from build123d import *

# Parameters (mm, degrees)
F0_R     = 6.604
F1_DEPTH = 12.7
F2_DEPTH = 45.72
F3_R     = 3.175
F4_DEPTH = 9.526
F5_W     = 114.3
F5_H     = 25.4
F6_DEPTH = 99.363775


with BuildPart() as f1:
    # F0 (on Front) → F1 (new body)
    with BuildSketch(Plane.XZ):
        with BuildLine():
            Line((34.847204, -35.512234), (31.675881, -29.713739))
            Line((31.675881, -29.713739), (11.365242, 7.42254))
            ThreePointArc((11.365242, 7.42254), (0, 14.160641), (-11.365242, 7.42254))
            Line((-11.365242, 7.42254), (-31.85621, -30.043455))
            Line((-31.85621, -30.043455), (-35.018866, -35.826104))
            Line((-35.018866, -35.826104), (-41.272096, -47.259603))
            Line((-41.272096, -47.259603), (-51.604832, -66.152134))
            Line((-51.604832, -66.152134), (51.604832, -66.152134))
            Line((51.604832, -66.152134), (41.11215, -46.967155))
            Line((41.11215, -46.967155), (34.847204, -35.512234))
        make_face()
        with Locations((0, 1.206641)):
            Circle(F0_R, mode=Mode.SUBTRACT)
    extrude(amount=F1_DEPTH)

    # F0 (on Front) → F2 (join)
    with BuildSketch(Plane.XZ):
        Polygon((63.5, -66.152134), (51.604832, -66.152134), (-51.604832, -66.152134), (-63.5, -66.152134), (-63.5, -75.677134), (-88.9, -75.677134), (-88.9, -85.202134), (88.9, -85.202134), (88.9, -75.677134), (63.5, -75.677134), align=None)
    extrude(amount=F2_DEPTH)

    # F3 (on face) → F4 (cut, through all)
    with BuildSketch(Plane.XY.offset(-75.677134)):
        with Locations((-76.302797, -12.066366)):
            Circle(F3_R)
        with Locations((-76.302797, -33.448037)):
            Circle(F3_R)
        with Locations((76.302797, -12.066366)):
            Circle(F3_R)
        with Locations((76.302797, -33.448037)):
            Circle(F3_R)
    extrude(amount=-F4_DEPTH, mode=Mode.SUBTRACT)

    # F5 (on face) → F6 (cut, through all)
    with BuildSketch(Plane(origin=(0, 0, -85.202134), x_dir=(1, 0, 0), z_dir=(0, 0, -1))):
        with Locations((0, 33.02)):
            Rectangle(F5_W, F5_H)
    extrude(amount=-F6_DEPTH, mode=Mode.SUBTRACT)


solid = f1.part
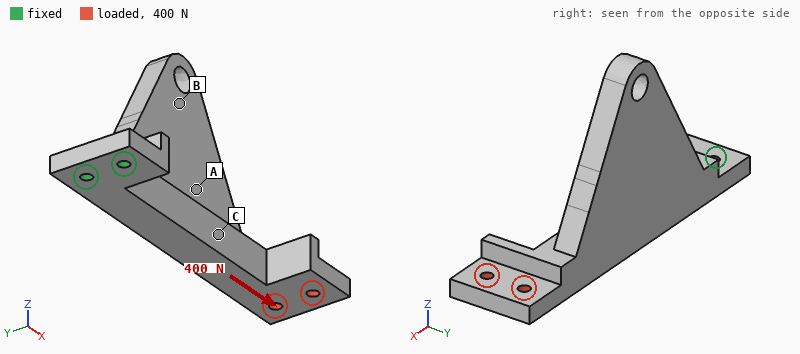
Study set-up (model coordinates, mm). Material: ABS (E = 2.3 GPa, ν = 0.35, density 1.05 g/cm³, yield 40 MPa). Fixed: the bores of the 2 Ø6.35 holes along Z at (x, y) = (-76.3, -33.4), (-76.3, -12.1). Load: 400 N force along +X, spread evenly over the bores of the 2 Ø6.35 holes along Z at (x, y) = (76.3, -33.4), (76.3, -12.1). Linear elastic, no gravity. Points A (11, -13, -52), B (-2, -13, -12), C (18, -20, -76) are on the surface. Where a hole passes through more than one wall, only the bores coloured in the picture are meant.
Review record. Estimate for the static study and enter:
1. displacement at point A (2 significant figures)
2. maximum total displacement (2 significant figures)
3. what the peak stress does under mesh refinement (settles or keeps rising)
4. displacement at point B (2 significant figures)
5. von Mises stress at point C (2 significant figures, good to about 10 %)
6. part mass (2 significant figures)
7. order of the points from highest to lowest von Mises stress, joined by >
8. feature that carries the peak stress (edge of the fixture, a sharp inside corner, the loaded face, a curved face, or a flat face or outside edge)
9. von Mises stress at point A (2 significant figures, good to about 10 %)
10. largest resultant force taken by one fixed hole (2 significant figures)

0.52 mm
2.0 mm
keeps rising
0.35 mm
3.8 MPa
140 g
C > A > B
a sharp inside corner
1.1 MPa
230 N
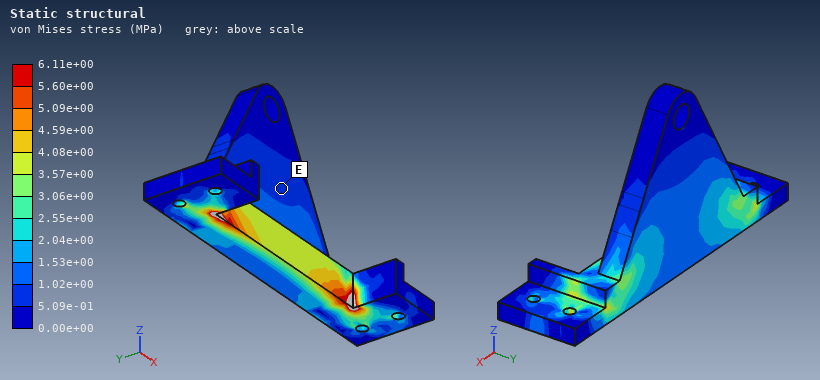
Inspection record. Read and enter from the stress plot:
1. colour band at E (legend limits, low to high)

5.09e-01 to 1.02e+00 MPa
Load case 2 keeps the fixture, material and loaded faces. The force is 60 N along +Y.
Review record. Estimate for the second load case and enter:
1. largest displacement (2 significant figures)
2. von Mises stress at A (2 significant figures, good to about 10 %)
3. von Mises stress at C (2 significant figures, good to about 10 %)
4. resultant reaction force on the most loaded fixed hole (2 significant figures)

2.5 mm
0.92 MPa
2.0 MPa
390 N
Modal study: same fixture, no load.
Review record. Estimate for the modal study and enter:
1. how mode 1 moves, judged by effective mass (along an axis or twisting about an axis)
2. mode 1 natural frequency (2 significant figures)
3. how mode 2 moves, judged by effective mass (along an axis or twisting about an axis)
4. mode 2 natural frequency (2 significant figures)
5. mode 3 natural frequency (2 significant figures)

along Z
84 Hz
along Y
140 Hz
270 Hz
